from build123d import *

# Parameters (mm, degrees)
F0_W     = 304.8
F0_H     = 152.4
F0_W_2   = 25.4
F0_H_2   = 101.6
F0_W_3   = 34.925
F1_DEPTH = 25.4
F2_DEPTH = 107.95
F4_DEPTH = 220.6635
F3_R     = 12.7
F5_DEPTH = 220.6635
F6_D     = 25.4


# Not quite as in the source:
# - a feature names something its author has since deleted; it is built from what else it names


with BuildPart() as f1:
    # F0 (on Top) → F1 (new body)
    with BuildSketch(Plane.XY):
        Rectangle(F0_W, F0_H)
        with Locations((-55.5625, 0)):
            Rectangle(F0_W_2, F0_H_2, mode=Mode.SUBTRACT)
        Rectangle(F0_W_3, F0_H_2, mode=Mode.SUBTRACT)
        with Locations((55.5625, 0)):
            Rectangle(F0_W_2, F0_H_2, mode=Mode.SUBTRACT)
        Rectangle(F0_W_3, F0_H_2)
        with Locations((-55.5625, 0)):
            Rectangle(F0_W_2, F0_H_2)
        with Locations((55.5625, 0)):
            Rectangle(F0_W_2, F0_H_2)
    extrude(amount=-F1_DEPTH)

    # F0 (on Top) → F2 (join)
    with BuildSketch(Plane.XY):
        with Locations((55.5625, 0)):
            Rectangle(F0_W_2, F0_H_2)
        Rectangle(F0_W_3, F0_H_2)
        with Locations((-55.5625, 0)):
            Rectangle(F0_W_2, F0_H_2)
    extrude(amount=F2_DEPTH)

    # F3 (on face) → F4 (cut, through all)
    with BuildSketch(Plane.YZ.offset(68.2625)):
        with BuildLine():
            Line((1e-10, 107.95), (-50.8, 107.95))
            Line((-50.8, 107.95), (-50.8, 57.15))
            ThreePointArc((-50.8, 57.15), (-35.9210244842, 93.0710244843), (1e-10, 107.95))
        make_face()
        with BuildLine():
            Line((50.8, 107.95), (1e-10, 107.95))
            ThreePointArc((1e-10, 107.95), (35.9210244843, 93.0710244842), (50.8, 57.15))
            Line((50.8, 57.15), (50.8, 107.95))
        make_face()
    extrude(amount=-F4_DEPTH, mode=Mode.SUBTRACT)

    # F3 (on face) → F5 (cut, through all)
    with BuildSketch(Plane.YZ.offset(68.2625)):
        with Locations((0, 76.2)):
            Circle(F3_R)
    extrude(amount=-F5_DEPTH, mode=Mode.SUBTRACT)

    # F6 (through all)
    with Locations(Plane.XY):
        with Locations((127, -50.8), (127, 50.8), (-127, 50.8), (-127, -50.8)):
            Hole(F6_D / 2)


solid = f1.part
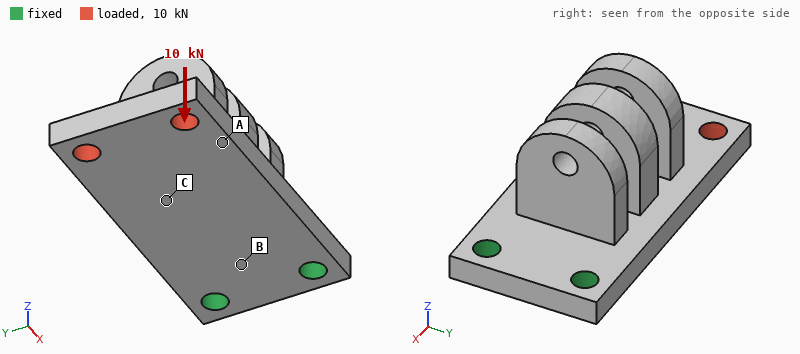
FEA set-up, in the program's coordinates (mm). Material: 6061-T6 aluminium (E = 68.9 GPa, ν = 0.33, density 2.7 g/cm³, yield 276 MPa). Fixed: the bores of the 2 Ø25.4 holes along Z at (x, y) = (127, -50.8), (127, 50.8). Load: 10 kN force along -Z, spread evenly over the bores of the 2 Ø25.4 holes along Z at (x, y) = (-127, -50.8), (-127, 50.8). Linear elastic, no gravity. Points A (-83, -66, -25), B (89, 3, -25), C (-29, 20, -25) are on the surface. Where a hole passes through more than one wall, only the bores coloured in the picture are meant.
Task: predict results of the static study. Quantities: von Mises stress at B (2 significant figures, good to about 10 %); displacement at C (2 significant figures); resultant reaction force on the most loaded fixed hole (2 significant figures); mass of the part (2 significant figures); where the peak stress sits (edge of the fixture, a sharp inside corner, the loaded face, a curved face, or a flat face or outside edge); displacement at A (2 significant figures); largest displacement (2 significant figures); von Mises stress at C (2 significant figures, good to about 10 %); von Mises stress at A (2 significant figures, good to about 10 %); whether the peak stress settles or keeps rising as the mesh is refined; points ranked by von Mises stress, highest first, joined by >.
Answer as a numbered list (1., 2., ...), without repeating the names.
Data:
1. 110 MPa
2. 1.5 mm
3. 5.1 kN
4. 5.2 kg
5. edge of the fixture
6. 2.4 mm
7. 3.8 mm
8. 58 MPa
9. 26 MPa
10. keeps rising
11. B > C > A
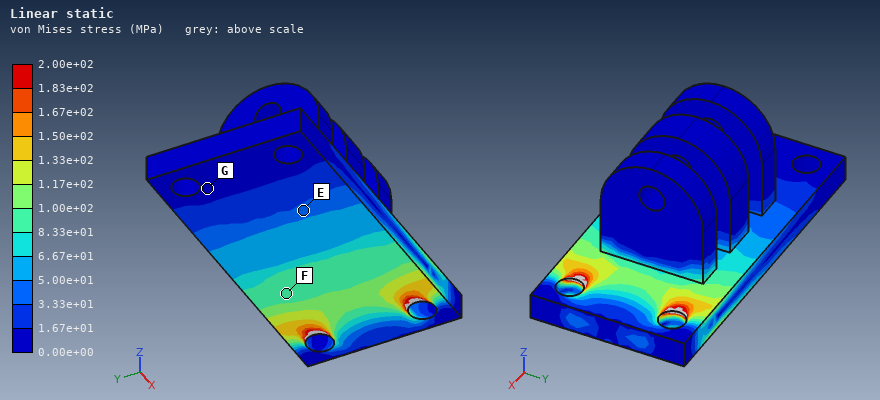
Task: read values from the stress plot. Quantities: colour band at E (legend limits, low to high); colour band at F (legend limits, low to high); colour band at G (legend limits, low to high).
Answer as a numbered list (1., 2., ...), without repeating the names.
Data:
1. 3.33e+01 to 5.00e+01 MPa
2. 8.33e+01 to 1.00e+02 MPa
3. 0.00e+00 to 1.67e+01 MPa
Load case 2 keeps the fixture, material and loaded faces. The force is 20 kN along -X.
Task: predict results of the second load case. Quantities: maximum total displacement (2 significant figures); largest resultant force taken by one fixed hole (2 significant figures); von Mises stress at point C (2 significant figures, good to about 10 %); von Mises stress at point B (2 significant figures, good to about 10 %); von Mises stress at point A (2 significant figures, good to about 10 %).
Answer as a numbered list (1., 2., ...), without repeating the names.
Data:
1. 31 µm
2. 10 kN
3. 4.8 MPa
4. 3.1 MPa
5. 6.8 MPa
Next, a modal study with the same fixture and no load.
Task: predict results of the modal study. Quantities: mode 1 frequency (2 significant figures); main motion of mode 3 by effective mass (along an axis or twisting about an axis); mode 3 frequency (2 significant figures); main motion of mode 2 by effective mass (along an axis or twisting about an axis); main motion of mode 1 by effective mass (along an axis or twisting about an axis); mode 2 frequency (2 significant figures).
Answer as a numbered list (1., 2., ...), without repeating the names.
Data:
1. 230 Hz
2. along Z
3. 1100 Hz
4. along Y
5. along Z
6. 750 Hz
